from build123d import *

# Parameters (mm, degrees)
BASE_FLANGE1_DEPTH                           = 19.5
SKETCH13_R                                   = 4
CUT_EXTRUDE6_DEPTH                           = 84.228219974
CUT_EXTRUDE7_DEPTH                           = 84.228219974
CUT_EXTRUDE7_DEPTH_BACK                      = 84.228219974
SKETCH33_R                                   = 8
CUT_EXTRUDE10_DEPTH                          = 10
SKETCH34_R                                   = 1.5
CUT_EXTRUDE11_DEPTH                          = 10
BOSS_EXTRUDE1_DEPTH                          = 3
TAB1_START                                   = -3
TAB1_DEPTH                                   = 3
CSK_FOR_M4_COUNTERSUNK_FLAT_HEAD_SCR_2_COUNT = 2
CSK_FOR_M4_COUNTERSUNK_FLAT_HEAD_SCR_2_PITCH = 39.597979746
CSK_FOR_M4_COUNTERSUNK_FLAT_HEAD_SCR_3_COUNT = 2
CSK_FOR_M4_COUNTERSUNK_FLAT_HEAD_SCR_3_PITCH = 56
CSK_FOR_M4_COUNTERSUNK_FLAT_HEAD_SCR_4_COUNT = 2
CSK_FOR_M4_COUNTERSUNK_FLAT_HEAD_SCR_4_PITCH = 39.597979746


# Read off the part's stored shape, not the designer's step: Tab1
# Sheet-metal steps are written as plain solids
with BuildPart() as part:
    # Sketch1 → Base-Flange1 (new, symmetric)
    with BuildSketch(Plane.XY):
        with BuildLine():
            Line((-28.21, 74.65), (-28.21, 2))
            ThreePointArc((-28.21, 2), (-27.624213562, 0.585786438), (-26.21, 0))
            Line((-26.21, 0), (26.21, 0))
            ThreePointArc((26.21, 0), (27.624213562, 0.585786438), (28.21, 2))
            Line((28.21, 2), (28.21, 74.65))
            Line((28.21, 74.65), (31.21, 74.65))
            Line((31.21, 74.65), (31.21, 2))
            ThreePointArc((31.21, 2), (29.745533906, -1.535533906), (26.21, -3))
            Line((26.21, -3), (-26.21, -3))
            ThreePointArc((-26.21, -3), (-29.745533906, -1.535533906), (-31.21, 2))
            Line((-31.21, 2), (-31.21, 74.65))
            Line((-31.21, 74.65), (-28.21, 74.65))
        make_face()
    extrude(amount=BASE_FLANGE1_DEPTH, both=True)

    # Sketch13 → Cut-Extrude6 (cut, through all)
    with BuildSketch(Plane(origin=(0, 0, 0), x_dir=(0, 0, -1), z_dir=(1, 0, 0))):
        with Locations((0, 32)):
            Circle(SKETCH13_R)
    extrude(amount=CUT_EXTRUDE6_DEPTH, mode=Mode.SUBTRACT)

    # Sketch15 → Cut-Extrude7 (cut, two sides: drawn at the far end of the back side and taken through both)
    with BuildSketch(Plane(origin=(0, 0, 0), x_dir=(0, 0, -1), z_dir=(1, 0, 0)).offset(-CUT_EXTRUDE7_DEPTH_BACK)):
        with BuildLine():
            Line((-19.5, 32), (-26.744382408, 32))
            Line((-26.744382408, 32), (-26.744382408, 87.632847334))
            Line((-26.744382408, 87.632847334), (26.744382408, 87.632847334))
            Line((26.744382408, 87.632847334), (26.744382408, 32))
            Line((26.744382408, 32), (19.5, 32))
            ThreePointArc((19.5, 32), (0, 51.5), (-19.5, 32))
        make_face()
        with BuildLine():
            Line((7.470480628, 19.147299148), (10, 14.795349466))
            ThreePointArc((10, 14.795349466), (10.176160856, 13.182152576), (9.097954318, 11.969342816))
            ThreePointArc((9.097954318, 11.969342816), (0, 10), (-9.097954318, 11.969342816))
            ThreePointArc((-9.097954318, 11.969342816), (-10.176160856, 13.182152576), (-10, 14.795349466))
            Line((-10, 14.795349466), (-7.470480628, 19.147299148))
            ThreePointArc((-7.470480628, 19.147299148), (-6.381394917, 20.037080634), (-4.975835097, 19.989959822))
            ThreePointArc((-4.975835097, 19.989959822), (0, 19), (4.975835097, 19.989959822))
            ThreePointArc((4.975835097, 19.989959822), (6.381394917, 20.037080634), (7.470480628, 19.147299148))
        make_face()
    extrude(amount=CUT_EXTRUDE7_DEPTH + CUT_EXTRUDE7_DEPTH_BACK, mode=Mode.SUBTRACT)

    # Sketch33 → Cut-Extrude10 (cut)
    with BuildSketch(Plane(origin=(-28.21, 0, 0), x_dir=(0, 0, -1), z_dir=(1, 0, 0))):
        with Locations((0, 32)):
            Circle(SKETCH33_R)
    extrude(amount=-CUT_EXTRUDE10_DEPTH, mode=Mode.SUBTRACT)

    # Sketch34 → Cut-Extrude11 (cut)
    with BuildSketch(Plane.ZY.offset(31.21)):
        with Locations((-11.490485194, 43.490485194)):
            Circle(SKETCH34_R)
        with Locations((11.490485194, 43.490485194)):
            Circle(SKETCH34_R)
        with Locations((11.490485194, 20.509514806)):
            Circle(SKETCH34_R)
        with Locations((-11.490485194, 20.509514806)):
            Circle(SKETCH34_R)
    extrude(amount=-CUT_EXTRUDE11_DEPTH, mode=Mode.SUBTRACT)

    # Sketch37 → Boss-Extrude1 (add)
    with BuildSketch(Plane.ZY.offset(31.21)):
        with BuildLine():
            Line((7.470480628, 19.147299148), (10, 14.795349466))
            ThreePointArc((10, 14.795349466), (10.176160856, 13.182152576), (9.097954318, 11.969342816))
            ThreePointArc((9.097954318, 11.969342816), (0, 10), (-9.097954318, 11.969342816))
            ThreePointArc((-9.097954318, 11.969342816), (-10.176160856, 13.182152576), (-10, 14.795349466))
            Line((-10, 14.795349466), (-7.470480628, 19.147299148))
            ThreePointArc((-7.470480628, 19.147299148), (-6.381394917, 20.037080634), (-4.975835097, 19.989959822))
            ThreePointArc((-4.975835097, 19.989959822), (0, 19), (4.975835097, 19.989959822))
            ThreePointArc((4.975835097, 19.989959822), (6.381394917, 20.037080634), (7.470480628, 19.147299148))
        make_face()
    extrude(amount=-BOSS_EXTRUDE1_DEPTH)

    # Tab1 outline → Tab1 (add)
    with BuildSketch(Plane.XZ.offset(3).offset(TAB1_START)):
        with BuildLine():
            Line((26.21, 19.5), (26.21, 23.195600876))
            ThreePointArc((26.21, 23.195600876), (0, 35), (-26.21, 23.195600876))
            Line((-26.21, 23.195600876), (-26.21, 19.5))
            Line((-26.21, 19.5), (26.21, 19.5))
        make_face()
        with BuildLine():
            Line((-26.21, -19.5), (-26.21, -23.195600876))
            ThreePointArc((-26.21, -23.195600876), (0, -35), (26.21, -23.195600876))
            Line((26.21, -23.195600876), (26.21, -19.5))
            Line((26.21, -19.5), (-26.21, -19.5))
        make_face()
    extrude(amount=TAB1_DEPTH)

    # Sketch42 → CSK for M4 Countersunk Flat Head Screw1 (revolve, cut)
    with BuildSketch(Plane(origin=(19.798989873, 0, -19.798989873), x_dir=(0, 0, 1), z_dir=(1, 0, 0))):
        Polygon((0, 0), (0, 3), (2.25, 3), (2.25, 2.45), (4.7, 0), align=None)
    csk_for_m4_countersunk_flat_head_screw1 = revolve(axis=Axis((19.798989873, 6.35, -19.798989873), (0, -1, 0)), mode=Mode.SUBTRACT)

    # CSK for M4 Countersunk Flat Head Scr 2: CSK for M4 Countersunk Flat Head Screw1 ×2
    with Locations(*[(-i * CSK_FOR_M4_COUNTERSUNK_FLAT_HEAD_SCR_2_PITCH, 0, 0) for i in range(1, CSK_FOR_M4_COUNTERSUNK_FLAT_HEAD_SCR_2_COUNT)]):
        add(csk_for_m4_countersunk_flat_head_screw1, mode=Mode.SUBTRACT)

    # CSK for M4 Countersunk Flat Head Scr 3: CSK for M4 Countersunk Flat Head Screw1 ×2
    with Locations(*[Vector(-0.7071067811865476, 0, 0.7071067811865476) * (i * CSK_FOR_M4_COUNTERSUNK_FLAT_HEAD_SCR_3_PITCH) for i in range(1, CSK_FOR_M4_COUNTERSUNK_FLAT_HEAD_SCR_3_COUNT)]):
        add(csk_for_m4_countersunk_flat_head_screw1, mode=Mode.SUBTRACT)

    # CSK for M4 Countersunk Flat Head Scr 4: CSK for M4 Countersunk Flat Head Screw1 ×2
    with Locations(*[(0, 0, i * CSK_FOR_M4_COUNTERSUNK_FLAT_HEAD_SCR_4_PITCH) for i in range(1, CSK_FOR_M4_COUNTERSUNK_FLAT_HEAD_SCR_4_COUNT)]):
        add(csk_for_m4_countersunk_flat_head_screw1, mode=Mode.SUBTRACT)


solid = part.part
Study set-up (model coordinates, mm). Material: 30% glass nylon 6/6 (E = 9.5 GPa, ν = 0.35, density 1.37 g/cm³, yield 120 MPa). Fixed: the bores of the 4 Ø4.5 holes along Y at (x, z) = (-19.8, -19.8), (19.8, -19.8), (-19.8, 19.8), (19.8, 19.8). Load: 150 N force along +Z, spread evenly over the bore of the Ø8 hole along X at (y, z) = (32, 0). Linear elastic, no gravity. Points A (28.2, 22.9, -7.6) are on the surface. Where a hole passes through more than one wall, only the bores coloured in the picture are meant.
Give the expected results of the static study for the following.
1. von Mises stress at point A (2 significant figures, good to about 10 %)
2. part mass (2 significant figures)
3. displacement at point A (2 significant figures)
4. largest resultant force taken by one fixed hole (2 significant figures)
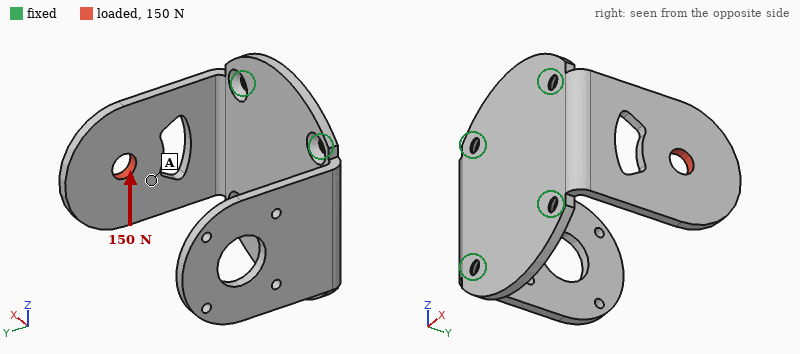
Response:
6.6 MPa
27 g
0.28 mm
200 N
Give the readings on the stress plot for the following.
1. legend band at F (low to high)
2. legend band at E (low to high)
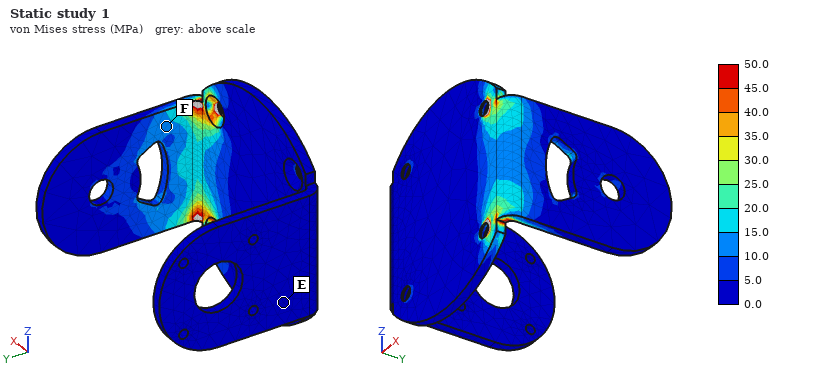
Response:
10.0 to 15.0 MPa
0.0 to 5.0 MPa
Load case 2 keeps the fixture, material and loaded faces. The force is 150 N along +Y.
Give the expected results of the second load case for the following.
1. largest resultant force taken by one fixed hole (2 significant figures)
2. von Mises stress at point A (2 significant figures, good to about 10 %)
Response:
150 N
3.1 MPa
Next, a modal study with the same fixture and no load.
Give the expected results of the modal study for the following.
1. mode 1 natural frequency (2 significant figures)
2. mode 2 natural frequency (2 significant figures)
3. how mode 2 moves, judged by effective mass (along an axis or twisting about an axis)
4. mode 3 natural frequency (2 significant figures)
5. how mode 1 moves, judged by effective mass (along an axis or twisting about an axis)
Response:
350 Hz
410 Hz
along X
1200 Hz
along X
